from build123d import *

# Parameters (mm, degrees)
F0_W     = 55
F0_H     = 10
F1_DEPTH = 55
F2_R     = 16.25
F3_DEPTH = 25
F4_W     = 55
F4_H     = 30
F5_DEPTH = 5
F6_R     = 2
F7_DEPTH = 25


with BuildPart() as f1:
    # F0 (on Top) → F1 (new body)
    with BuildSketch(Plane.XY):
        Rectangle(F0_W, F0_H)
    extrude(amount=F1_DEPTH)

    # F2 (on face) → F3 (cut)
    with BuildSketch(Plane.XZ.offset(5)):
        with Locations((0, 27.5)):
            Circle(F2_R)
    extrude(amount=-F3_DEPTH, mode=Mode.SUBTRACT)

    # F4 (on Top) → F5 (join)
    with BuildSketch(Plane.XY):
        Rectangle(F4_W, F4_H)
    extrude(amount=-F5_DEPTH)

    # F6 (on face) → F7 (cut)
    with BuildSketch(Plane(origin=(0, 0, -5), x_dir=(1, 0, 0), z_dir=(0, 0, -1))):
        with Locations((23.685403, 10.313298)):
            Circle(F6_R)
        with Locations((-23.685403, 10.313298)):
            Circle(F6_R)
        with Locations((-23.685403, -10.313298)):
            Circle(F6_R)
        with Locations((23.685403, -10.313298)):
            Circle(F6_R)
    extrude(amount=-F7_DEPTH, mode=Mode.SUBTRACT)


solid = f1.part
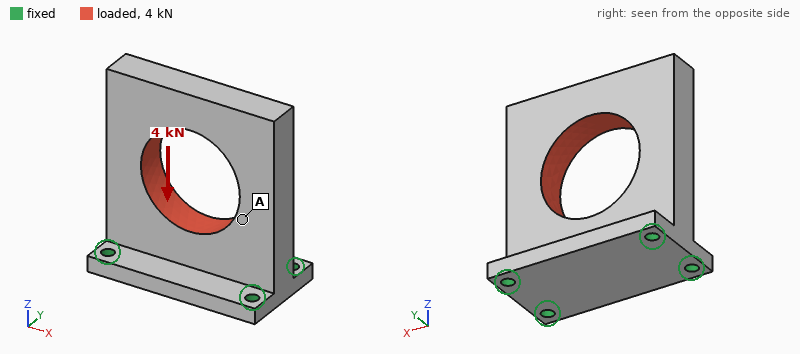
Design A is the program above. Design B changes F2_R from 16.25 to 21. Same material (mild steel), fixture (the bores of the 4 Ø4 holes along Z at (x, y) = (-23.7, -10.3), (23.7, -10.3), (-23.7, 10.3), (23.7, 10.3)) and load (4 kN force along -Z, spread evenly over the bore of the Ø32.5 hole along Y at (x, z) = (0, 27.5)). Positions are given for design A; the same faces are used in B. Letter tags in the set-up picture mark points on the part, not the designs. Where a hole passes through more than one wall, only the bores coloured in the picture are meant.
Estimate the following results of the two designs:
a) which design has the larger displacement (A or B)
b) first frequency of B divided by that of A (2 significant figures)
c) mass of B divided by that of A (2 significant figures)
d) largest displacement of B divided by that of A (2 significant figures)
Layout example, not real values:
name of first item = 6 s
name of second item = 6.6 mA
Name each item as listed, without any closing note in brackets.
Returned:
which design has the larger displacement = B
first frequency of B divided by that of A = 0.96
mass of B divided by that of A = 0.81
largest displacement of B divided by that of A = 2.1
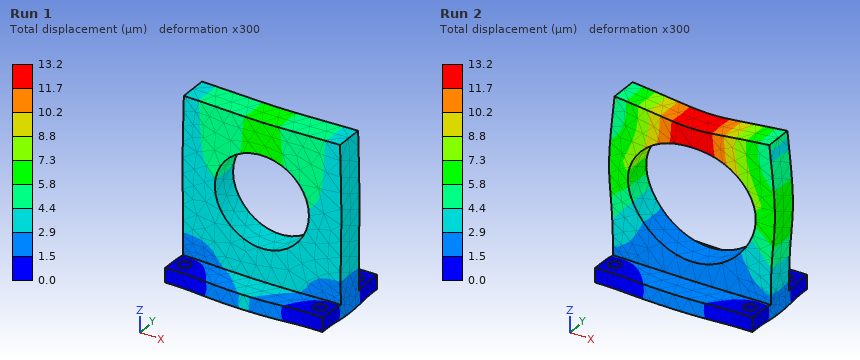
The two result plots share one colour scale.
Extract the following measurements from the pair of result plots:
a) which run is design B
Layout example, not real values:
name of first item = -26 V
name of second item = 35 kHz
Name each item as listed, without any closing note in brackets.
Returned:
which run is design B = Run 2
